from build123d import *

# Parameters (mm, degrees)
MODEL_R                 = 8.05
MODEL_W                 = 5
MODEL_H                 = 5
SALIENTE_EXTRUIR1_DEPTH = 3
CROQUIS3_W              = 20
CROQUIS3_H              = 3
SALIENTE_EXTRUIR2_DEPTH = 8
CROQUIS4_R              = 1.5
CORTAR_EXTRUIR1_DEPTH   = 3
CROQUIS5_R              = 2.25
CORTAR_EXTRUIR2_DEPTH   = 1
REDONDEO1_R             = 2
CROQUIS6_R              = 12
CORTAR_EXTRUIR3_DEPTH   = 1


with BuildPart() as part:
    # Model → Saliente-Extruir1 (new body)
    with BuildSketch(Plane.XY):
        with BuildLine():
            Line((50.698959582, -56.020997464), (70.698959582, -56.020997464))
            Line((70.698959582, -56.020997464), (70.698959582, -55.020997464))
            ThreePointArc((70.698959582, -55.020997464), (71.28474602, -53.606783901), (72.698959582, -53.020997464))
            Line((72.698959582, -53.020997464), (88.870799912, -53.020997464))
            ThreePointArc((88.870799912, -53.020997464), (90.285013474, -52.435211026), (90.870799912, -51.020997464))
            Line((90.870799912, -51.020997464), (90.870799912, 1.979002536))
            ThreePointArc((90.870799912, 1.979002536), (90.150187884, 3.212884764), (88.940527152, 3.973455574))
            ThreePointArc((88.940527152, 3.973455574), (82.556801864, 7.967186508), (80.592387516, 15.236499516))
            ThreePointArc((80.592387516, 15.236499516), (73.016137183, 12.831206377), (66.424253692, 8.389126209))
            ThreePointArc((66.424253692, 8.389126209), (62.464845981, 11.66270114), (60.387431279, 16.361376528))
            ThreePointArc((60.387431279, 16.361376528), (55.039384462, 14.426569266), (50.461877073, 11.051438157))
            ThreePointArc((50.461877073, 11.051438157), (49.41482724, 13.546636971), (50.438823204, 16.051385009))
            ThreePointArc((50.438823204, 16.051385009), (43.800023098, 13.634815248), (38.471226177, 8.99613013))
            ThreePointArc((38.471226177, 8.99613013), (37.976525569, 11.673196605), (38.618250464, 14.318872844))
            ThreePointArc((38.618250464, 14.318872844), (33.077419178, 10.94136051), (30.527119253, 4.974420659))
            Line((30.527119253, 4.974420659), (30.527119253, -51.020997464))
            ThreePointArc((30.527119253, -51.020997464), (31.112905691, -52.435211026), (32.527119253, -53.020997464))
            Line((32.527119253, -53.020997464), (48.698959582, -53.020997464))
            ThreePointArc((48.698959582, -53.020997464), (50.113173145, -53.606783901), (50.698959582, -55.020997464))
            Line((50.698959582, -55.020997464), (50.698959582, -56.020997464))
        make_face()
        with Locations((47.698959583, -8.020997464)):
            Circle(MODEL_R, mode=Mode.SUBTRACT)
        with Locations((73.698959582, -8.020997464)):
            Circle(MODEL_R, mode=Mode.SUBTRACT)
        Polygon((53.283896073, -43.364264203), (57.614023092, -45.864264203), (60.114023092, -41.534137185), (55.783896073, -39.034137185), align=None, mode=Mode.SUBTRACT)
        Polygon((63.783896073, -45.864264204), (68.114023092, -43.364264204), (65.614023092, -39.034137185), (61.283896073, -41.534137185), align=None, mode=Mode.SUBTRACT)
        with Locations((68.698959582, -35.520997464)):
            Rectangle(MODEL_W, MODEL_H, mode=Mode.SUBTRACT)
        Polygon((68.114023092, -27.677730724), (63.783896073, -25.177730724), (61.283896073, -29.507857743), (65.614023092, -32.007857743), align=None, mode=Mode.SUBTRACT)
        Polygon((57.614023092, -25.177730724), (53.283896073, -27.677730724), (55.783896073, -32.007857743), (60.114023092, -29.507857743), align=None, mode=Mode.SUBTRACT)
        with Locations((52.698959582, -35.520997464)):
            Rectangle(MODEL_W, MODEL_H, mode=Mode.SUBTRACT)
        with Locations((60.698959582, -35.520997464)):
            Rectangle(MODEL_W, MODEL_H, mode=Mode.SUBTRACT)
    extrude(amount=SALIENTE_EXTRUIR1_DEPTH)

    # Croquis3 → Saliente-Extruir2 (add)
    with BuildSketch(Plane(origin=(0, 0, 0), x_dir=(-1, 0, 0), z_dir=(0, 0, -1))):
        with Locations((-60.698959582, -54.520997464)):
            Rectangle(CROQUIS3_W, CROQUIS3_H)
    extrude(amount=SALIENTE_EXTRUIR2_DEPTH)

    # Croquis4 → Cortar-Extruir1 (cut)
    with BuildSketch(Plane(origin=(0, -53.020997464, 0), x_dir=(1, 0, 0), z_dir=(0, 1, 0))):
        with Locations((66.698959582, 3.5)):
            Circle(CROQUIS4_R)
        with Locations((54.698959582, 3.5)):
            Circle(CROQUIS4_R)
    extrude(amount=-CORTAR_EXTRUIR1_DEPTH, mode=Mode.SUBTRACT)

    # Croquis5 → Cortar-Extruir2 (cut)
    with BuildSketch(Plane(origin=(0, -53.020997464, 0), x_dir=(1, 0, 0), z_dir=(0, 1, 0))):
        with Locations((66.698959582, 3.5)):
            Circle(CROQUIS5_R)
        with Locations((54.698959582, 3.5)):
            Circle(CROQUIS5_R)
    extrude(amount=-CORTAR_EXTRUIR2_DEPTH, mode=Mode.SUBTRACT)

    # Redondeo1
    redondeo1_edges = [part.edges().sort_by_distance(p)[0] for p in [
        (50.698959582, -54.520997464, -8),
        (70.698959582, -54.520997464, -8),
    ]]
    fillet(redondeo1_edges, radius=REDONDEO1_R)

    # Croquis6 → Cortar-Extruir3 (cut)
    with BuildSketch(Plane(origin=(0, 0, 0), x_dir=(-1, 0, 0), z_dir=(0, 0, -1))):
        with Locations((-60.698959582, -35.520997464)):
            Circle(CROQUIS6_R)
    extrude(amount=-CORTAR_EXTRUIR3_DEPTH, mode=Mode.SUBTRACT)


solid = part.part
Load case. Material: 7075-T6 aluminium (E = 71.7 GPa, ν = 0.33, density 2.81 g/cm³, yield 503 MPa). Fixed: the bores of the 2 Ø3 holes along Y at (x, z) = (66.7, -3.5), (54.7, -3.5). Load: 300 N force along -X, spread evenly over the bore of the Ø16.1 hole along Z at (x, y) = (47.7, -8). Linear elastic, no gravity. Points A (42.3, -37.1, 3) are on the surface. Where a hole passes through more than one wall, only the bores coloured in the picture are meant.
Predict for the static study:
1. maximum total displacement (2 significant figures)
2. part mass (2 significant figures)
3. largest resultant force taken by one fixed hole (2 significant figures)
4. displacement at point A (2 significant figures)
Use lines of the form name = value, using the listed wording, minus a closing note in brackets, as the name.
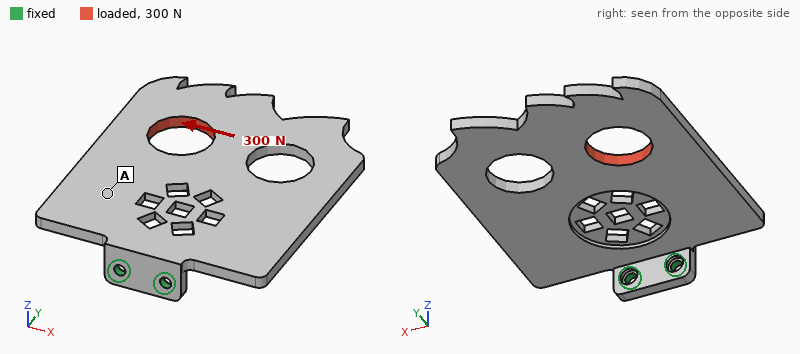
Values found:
maximum total displacement = 0.38 mm
part mass = 29 g
largest resultant force taken by one fixed hole = 1.1 kN
displacement at point A = 0.14 mm
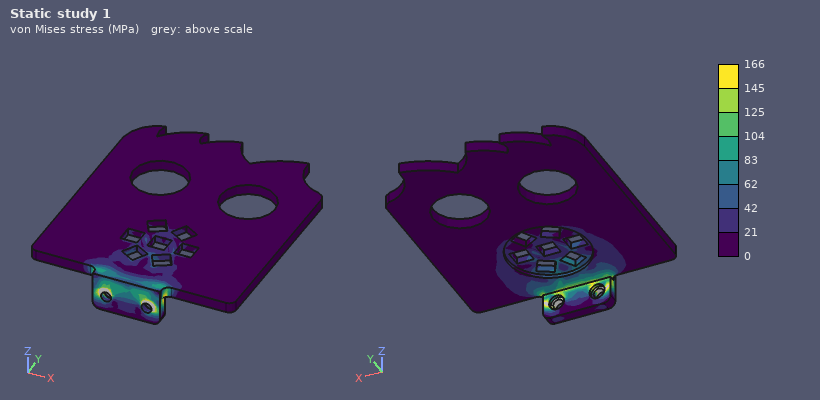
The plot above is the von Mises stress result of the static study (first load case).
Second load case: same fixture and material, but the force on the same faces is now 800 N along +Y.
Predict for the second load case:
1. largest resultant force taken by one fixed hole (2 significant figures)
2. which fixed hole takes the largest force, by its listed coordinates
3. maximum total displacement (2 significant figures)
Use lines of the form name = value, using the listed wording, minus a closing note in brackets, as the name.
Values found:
largest resultant force taken by one fixed hole = 1.2 kN
which fixed hole takes the largest force, by its listed coordinates = (54.7, -3.5)
maximum total displacement = 0.45 mm
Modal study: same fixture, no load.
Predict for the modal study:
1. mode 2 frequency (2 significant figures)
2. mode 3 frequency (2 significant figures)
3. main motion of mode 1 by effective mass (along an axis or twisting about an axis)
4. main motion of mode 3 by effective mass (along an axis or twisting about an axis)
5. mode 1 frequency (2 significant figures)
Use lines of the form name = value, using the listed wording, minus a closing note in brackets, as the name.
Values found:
mode 2 frequency = 870 Hz
mode 3 frequency = 1300 Hz
main motion of mode 1 by effective mass = along Z
main motion of mode 3 by effective mass = along X
mode 1 frequency = 340 Hz
